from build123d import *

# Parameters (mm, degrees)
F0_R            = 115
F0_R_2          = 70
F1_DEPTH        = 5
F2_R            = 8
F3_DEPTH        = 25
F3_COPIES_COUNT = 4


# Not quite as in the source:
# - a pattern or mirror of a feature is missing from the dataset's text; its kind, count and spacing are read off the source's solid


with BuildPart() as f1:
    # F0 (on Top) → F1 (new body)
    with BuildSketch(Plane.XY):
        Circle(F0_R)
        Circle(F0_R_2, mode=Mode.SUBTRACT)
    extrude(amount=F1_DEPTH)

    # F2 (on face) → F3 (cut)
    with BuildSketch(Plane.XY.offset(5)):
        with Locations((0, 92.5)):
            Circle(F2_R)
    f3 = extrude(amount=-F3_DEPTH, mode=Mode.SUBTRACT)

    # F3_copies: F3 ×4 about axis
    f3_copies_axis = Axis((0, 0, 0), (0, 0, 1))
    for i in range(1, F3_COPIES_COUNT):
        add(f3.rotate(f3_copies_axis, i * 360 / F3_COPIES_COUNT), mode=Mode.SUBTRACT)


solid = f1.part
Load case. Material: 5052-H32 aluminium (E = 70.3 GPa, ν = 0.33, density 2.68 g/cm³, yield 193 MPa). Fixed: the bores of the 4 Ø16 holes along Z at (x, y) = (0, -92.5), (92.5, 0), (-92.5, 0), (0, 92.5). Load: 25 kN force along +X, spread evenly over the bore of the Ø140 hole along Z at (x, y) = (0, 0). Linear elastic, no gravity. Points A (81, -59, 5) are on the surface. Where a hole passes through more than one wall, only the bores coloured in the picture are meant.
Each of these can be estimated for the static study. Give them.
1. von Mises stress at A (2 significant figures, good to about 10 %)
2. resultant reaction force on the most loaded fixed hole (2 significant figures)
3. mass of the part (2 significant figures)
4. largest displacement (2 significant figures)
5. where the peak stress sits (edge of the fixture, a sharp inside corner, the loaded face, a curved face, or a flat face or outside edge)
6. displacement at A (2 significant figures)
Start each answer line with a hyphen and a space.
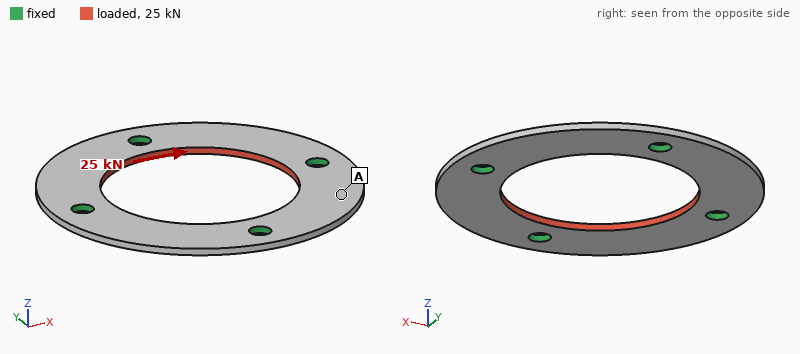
- 11 MPa
- 7.5 kN
- 340 g
- 26 µm
- edge of the fixture
- 22 µm
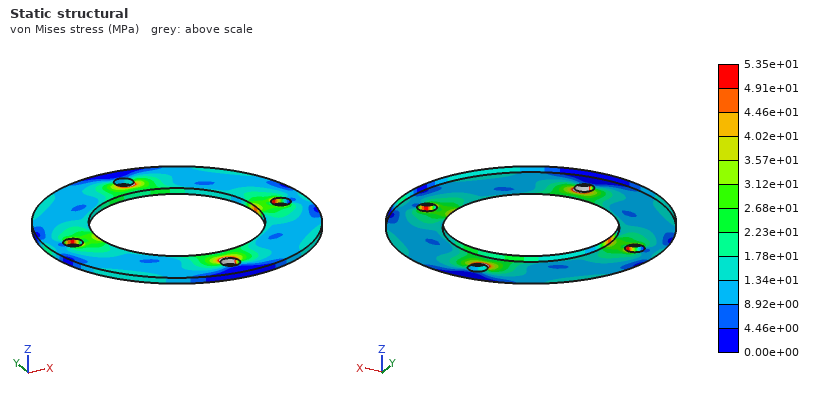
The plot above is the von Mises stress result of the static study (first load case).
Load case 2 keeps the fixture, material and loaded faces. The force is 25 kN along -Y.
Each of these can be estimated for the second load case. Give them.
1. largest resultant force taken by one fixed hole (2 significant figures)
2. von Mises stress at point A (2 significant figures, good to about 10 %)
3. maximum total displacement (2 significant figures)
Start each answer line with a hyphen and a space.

- 7.5 kN
- 12 MPa
- 26 µm
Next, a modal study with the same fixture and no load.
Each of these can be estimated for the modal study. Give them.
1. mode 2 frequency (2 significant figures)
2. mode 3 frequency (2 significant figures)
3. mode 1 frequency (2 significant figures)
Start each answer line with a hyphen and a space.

- 1300 Hz
- 1300 Hz
- 1300 Hz
